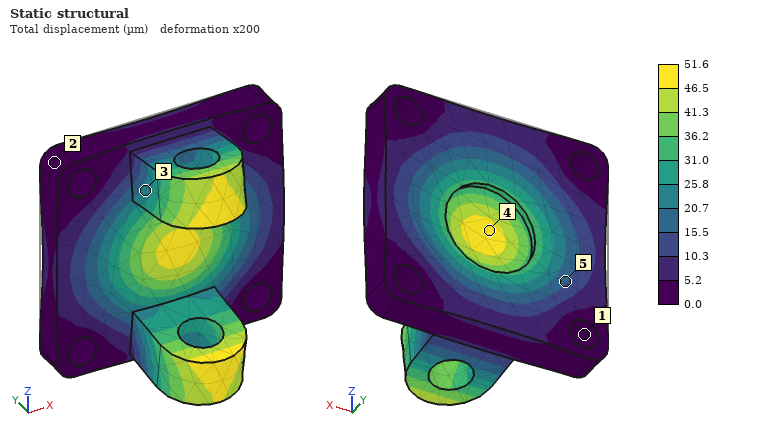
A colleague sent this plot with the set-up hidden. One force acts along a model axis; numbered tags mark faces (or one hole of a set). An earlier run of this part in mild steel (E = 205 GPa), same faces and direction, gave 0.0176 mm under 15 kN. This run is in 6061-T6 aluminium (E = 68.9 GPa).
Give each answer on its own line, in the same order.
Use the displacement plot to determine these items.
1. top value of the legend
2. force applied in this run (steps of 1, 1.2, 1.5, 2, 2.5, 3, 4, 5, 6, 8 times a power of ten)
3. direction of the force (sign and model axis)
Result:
51.6 µm
15 kN
-Y
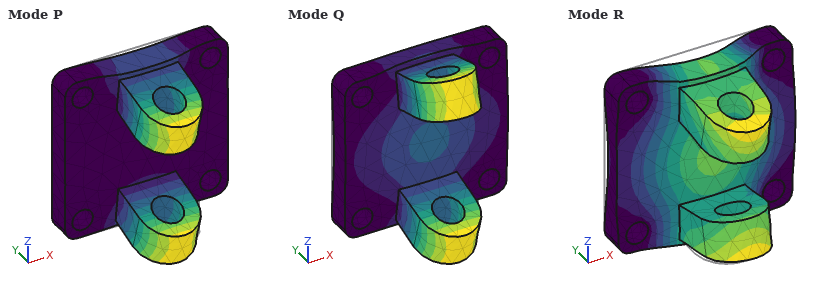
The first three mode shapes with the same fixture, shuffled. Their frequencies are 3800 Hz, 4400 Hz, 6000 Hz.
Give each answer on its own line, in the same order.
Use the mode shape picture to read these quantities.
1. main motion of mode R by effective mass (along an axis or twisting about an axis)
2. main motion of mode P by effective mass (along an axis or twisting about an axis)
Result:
along Y
along Z
